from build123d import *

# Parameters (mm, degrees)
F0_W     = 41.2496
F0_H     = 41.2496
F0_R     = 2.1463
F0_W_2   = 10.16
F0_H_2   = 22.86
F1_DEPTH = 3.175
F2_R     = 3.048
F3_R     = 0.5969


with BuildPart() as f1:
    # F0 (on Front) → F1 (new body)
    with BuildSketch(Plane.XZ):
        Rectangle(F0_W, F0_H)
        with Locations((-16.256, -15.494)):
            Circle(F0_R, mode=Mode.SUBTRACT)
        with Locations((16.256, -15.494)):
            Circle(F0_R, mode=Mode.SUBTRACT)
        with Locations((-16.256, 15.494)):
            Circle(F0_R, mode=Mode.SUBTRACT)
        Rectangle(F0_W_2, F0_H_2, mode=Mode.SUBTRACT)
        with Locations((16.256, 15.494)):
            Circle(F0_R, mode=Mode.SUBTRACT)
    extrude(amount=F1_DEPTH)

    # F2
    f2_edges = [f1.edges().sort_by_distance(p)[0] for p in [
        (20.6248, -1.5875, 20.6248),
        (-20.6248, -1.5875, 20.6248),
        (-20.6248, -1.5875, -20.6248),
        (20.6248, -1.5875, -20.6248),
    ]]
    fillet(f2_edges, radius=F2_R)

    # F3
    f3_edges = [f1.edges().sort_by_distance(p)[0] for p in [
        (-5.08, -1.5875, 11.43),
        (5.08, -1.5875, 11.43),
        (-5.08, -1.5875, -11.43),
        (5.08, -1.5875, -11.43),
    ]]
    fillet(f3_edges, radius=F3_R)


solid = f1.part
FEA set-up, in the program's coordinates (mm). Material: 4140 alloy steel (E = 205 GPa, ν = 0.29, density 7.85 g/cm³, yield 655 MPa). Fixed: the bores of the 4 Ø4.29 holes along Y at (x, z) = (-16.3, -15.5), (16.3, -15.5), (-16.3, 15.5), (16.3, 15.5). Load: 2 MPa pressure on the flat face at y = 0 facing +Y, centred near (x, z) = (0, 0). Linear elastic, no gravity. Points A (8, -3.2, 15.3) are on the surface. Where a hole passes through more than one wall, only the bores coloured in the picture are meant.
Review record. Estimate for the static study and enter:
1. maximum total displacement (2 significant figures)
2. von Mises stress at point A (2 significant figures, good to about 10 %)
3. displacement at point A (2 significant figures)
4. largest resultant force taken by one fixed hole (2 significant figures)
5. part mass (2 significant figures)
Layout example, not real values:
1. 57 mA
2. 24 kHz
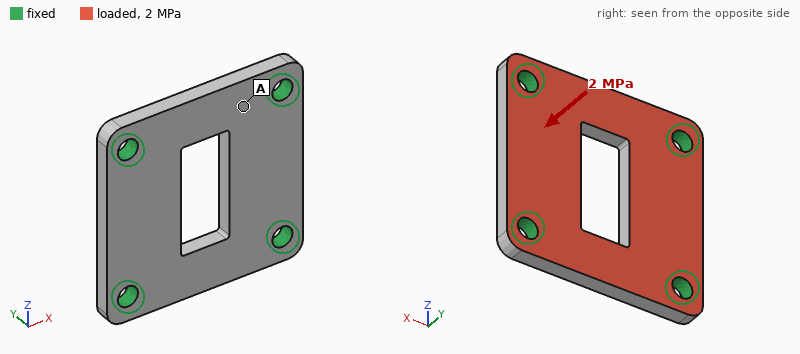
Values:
1. 19 µm
2. 25 MPa
3. 6.1 µm
4. 700 N
5. 35 g
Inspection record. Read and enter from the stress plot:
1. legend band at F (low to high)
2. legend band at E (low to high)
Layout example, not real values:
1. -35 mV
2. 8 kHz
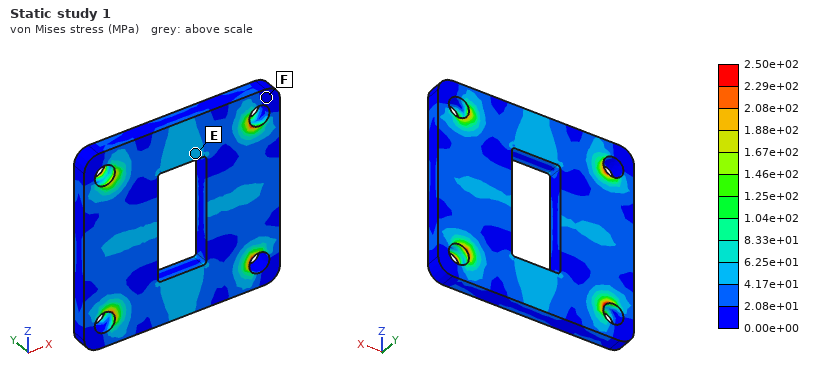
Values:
1. 0.00e+00 to 2.08e+01 MPa
2. 4.17e+01 to 6.25e+01 MPa
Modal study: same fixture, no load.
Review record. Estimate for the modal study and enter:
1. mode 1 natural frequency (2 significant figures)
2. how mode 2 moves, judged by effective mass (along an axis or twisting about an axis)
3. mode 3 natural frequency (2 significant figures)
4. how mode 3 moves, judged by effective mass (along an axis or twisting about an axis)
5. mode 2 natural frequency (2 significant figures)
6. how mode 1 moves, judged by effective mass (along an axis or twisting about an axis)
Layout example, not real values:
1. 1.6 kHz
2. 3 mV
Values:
1. 14 kHz
2. twisting about Z
3. 19 kHz
4. twisting about X
5. 17 kHz
6. along Y
